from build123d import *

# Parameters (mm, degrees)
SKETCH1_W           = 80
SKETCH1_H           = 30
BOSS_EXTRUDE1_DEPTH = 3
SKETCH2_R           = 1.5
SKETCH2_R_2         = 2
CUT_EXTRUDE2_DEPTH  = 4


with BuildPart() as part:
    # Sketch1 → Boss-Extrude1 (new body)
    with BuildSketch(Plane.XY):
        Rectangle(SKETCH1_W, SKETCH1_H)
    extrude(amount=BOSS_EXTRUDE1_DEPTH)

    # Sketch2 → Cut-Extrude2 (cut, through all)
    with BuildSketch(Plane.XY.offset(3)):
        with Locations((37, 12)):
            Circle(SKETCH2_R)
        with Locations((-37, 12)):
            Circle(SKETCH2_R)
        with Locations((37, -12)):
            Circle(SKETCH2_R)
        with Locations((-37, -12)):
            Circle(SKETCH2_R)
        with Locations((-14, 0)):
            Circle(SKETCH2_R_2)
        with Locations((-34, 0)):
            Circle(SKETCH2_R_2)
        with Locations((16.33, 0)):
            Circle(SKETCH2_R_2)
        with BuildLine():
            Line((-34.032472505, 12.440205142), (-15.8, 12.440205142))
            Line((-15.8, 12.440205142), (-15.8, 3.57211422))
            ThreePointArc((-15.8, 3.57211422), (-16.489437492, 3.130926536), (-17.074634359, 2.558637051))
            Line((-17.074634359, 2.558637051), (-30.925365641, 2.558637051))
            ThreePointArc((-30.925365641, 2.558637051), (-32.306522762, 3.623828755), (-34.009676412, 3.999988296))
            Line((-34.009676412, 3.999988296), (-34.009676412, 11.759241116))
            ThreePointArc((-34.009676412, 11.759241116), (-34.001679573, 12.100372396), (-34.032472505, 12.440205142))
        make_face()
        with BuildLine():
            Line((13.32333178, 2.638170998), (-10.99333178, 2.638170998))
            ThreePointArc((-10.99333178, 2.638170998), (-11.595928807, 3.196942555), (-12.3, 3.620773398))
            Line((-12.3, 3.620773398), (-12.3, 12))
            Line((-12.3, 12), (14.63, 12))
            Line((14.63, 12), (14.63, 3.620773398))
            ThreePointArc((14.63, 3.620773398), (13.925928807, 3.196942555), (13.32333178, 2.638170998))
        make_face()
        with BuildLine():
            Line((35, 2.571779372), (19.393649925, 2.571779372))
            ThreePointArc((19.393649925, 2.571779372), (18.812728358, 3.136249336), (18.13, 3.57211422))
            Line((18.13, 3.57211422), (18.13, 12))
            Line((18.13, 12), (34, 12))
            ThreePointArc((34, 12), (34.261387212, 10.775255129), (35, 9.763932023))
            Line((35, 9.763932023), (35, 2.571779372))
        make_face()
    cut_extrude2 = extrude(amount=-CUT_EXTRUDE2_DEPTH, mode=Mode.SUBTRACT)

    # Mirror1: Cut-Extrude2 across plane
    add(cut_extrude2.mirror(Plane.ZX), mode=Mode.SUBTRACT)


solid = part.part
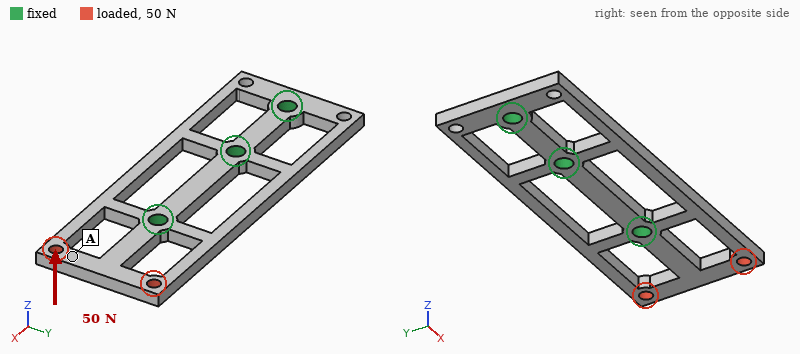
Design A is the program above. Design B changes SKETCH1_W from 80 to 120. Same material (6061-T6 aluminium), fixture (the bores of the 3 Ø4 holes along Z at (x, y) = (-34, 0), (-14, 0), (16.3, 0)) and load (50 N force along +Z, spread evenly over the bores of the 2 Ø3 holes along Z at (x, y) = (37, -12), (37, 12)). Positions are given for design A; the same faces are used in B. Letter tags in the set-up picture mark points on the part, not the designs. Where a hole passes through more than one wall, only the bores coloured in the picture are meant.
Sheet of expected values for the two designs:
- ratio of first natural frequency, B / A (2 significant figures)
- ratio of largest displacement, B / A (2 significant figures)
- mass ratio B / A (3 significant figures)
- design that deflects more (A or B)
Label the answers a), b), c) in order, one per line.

a) 0.27
b) 1.9
c) 2.03
d) B
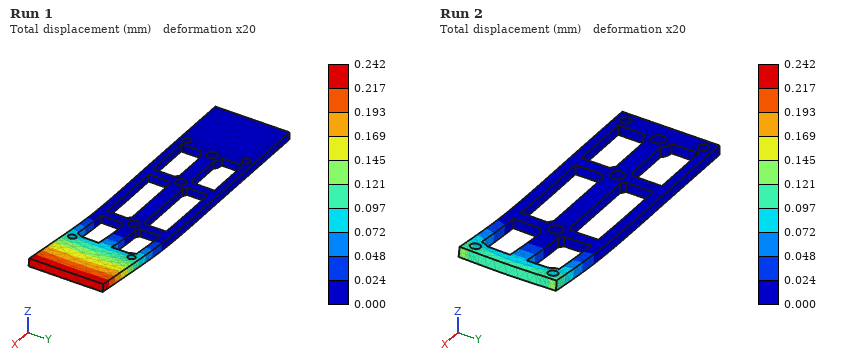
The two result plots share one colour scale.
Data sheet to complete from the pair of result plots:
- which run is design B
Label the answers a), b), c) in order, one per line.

a) Run 1
